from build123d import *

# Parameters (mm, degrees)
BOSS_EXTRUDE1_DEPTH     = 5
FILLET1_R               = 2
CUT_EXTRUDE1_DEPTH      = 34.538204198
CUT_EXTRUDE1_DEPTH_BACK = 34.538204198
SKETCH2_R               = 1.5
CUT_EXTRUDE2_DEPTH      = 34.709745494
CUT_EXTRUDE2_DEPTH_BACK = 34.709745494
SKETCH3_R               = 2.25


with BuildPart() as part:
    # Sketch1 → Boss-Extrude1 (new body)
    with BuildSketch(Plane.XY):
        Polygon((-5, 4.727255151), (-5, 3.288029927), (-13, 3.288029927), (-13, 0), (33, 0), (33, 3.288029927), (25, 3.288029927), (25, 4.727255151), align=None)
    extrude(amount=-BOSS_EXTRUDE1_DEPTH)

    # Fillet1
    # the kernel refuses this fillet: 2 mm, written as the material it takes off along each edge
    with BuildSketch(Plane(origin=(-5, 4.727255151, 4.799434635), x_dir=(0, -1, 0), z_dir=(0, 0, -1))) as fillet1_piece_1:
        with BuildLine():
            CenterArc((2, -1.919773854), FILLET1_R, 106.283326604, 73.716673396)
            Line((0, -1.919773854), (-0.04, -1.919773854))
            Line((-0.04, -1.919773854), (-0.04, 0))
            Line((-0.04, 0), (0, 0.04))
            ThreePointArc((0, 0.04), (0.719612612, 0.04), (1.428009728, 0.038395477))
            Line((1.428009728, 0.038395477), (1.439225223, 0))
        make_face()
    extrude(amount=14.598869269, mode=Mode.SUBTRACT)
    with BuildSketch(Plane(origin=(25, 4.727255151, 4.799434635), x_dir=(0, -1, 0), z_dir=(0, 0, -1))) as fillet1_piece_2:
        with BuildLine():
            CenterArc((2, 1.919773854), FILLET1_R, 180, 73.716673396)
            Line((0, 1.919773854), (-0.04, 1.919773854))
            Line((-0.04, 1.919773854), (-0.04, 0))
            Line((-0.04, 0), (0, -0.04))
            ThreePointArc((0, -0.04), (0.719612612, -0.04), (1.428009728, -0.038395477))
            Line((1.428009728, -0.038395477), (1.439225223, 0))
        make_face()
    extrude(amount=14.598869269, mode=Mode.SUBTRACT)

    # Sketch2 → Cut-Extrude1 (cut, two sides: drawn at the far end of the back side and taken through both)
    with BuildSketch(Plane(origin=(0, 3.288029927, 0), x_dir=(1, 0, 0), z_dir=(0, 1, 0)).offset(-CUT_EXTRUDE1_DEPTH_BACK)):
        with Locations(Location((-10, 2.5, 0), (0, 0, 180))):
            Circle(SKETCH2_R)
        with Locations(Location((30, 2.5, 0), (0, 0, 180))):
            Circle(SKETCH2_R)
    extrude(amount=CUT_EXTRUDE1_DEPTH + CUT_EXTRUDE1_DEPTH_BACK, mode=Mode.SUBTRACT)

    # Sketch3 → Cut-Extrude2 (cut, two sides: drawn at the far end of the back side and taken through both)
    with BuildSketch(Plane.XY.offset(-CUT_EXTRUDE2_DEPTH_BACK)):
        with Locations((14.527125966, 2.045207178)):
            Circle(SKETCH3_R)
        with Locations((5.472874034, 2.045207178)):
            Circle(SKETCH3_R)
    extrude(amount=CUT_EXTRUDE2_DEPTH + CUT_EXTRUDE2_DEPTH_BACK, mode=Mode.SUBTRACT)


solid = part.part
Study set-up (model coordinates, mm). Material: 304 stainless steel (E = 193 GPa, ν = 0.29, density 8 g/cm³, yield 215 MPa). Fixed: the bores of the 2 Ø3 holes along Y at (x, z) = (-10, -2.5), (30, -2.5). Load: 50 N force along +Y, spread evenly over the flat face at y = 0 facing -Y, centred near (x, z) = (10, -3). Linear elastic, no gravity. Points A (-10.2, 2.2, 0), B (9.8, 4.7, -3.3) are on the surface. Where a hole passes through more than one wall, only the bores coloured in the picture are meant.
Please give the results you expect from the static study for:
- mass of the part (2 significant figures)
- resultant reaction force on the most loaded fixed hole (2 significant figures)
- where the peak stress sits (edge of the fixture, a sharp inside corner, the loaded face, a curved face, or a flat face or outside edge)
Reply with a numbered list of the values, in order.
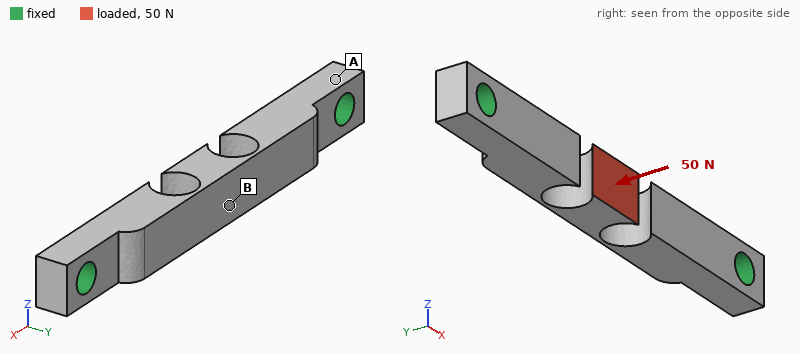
1. 6.1 g
2. 57 N
3. a curved face
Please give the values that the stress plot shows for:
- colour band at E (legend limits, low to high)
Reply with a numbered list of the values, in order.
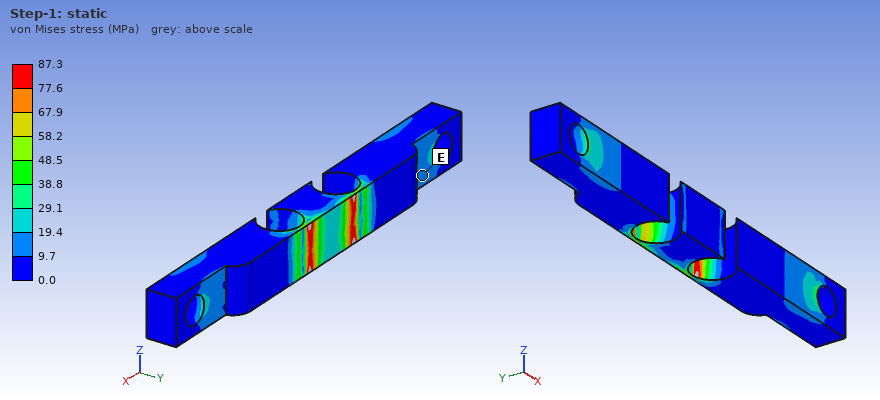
1. 9.7 to 19.4 MPa
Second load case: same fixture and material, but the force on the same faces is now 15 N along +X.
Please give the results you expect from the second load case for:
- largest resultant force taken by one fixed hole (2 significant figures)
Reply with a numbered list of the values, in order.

1. 9.9 N
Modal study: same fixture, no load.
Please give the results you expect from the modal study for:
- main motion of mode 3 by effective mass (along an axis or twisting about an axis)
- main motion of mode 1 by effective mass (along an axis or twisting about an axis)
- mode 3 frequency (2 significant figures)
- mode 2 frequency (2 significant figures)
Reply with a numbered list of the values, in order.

1. along Y
2. along Z
3. 11 kHz
4. 10 kHz
